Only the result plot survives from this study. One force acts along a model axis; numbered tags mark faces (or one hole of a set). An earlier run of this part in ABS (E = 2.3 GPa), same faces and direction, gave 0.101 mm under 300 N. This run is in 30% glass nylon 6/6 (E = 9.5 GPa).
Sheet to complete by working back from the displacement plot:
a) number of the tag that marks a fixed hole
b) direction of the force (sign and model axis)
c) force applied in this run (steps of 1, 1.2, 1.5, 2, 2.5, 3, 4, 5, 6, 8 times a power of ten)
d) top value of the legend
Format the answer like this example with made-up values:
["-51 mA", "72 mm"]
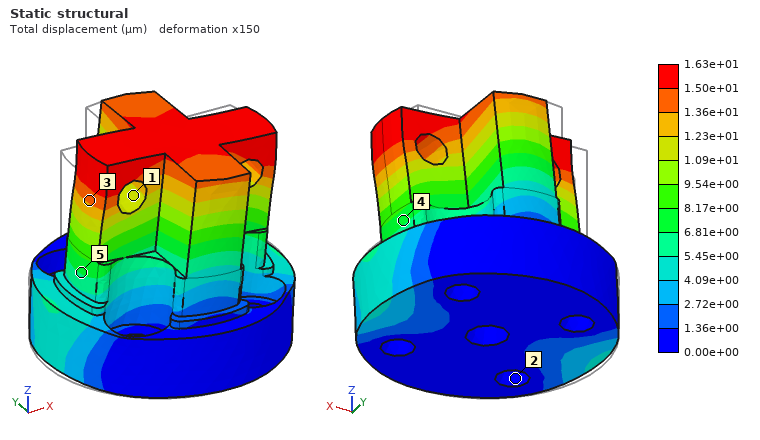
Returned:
["2", "+X", "200 N", "1.63e+01 µm"]
